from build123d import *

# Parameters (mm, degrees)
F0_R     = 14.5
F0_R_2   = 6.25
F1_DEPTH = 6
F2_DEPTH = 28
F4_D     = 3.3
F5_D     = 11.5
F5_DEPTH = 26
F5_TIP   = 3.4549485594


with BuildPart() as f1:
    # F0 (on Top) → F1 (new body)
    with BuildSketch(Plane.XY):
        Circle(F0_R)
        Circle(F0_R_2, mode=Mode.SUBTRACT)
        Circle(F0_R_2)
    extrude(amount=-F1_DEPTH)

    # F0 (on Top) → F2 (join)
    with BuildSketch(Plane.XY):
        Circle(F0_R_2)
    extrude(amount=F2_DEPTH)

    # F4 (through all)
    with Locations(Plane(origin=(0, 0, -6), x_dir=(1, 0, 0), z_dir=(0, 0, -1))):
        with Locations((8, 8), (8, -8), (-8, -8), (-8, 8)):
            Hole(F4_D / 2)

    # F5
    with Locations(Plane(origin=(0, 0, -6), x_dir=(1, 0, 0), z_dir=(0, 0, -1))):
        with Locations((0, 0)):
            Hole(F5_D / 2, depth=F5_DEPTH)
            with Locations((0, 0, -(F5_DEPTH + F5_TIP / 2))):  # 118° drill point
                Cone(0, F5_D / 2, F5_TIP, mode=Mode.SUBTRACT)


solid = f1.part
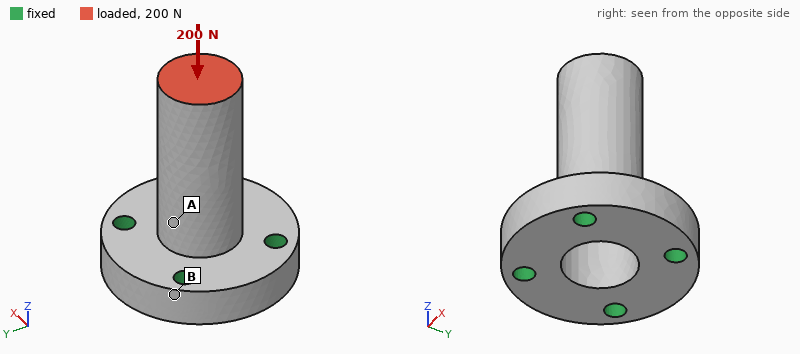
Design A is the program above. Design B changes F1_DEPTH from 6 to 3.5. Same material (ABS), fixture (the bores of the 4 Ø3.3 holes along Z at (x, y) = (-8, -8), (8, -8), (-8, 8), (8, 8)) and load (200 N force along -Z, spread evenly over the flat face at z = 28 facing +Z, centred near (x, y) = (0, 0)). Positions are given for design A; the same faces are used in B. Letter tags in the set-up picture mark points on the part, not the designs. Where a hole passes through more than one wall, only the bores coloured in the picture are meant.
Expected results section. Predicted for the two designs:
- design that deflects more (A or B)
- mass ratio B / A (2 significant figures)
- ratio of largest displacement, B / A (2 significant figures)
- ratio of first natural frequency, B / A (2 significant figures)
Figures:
B
0.70
1.1
0.92
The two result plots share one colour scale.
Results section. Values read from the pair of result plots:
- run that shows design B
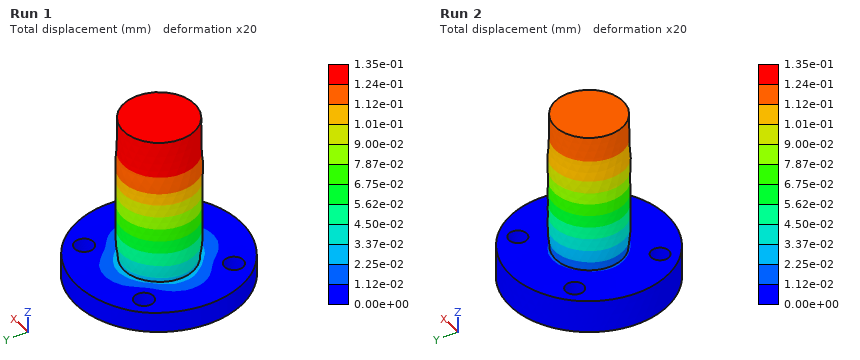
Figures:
Run 1
